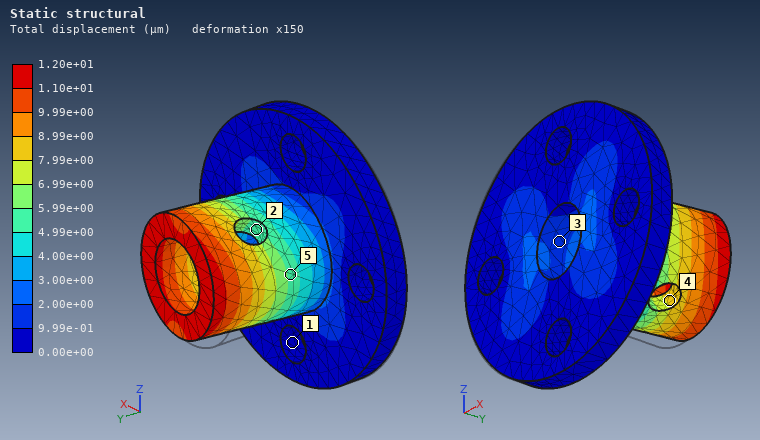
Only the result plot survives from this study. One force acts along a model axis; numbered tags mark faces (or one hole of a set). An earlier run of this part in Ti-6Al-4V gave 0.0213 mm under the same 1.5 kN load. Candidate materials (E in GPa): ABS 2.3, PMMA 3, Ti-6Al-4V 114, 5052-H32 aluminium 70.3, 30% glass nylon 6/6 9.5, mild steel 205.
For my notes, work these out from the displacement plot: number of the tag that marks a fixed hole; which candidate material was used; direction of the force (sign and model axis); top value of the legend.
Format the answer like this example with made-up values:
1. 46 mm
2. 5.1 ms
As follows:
1. 1
2. mild steel
3. +X
4. 1.20e+01 µm
